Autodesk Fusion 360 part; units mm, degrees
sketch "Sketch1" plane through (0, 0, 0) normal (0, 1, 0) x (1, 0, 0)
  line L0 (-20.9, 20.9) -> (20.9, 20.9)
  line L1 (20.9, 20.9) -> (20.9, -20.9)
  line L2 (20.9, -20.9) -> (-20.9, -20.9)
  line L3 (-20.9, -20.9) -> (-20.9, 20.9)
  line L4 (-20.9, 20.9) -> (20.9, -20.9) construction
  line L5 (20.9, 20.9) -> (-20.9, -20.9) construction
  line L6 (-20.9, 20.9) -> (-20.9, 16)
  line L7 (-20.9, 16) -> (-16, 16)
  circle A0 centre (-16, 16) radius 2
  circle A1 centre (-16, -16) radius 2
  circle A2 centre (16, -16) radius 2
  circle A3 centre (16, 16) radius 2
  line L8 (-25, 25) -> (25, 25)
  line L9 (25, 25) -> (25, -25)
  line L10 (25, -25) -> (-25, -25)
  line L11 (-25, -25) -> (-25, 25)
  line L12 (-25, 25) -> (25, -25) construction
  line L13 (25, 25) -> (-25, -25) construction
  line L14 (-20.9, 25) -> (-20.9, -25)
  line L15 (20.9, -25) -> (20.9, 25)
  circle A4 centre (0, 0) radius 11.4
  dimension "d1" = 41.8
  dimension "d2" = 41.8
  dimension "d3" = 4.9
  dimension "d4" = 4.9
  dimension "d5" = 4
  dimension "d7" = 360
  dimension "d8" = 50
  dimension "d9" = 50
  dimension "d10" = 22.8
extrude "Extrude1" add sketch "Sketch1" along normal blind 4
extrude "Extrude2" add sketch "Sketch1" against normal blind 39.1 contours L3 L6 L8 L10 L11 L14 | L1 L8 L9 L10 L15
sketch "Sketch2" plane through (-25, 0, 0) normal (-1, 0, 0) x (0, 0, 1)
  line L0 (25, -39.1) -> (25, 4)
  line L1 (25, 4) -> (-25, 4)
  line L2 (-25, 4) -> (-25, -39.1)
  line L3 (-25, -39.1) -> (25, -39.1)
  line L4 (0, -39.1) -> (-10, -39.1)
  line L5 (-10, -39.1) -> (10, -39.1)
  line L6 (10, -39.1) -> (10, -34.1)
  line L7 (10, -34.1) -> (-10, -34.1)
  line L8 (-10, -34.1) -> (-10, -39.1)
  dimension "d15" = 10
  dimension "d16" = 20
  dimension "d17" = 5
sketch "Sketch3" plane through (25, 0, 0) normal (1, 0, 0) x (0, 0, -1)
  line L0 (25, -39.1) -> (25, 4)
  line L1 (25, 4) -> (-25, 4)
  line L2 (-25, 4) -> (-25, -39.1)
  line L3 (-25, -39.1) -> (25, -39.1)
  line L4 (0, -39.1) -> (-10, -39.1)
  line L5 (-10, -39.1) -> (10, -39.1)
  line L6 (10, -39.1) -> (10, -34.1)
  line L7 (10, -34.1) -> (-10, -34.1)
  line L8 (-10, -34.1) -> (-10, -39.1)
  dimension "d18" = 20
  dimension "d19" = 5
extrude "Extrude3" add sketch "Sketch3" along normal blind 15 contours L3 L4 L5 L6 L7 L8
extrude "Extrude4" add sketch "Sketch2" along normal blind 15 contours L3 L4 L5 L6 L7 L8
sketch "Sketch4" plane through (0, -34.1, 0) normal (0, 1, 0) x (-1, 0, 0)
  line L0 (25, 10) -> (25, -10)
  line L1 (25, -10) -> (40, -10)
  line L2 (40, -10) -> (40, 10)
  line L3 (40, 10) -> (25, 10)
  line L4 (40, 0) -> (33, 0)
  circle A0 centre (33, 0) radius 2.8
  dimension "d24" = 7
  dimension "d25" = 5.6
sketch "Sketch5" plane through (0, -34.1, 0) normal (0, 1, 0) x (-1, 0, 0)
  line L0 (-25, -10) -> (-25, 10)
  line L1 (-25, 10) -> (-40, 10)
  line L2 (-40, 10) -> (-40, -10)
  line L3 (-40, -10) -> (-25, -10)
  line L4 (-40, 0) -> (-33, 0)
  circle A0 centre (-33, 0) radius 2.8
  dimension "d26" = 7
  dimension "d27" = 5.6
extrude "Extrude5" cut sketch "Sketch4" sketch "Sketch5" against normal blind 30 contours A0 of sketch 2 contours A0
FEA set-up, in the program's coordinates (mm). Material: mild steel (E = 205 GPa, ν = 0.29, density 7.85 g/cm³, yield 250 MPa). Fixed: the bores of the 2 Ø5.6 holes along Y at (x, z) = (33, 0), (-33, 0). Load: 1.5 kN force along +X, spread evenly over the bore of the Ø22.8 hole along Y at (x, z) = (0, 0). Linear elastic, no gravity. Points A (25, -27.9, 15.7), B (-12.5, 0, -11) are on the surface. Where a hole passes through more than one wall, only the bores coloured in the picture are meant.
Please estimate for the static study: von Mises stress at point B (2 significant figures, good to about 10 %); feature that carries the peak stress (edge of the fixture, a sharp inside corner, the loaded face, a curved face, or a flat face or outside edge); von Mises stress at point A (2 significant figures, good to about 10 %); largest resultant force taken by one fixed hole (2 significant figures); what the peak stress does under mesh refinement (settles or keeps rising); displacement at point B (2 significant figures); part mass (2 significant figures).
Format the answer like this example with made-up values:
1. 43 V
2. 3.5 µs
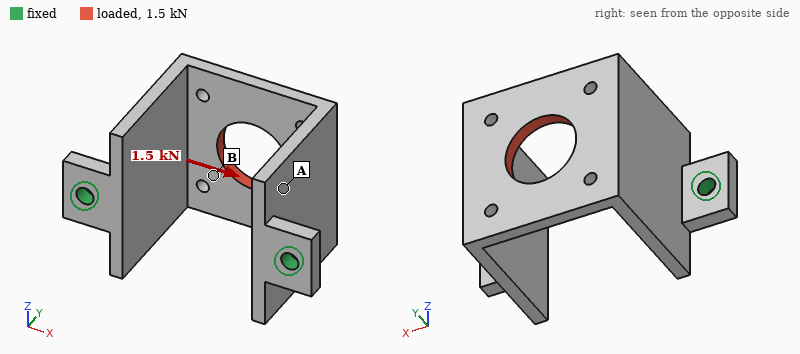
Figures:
1. 96 MPa
2. edge of the fixture
3. 39 MPa
4. 1.0 kN
5. keeps rising
6. 0.15 mm
7. 210 g
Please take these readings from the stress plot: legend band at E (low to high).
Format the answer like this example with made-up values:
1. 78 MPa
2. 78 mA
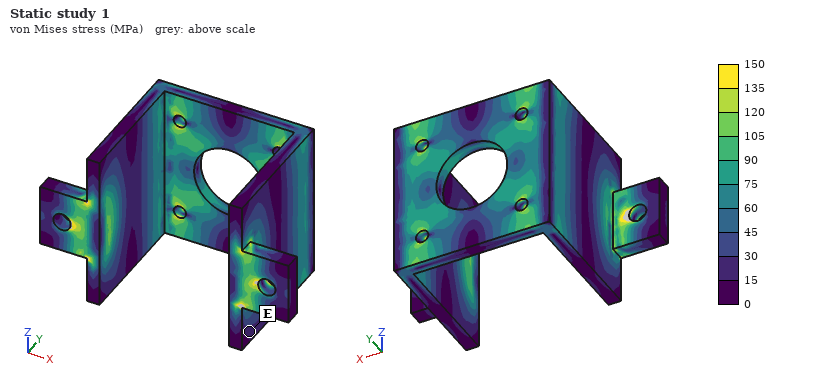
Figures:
1. 15 to 30 MPa
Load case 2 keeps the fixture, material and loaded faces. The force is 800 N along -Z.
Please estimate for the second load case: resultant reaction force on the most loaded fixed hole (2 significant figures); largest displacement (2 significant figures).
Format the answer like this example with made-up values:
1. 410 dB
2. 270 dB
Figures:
1. 400 N
2. 92 µm
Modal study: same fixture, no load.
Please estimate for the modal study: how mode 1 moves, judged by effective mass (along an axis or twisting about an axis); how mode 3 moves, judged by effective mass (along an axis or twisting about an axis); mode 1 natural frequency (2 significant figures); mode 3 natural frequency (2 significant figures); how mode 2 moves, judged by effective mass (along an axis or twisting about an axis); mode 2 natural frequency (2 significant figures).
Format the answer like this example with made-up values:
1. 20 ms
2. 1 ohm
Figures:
1. along Z
2. twisting about Y
3. 1500 Hz
4. 2100 Hz
5. along X
6. 1600 Hz
